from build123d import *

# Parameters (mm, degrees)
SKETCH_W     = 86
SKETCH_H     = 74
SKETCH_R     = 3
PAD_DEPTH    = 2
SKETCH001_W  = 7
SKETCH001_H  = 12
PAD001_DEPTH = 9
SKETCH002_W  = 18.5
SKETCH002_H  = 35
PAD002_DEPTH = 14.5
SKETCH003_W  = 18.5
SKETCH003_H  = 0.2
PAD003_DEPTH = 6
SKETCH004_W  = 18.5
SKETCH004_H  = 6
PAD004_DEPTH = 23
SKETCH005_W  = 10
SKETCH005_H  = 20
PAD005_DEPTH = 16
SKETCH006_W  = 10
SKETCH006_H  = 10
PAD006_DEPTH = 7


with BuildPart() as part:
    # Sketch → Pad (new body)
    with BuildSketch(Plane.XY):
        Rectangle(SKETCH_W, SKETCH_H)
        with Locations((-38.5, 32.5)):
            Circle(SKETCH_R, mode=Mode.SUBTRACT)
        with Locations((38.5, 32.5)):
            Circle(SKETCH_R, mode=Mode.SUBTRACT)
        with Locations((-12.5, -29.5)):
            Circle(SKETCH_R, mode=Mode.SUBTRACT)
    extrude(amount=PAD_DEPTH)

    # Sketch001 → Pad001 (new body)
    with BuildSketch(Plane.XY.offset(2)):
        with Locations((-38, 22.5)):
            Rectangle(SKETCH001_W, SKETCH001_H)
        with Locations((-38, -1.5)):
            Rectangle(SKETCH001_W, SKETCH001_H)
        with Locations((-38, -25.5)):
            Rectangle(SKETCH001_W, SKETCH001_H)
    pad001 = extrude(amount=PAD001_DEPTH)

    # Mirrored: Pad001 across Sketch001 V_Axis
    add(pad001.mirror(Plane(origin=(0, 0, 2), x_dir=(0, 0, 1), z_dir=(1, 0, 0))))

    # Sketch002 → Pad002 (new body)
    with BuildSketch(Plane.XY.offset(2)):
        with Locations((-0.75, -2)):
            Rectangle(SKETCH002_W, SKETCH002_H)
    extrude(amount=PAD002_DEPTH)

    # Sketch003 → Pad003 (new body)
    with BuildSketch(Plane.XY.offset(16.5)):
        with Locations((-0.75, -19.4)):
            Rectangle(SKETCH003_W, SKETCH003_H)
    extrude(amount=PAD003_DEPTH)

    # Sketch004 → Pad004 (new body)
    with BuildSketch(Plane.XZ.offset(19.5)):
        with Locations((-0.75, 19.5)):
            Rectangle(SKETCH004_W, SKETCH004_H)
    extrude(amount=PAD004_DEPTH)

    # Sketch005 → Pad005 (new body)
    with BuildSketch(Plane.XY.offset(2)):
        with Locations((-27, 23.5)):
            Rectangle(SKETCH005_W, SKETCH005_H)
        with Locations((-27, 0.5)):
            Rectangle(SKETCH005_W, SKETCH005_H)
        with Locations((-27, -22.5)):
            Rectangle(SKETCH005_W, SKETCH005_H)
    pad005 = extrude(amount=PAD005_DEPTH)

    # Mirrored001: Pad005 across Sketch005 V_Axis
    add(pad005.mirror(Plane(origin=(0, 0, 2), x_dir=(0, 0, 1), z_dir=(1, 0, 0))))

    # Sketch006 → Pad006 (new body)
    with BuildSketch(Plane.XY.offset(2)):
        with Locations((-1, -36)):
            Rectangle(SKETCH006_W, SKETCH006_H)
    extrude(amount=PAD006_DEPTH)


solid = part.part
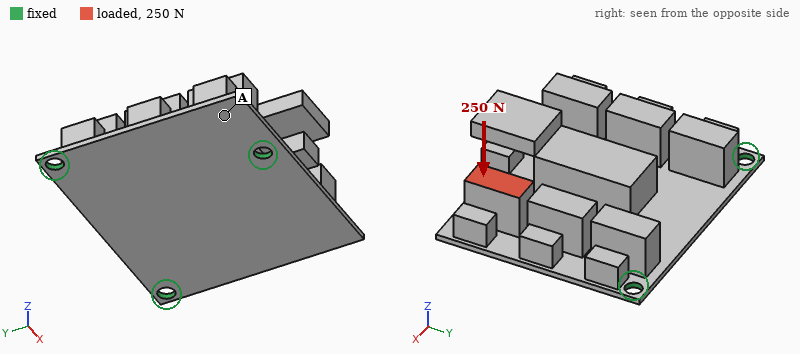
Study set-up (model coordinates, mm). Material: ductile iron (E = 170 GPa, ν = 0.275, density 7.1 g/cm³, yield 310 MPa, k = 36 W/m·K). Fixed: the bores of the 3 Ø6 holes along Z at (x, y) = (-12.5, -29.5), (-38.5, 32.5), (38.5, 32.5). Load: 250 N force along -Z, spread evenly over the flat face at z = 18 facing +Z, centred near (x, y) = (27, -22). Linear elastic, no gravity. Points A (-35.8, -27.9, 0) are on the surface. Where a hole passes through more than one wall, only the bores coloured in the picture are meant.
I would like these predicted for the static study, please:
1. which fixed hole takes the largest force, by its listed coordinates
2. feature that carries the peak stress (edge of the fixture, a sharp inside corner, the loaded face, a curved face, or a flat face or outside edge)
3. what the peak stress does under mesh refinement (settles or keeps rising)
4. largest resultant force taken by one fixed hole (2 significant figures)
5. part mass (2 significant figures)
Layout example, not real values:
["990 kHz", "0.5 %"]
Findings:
["(-12.5, -29.5)", "edge of the fixture", "keeps rising", "230 N", "350 g"]
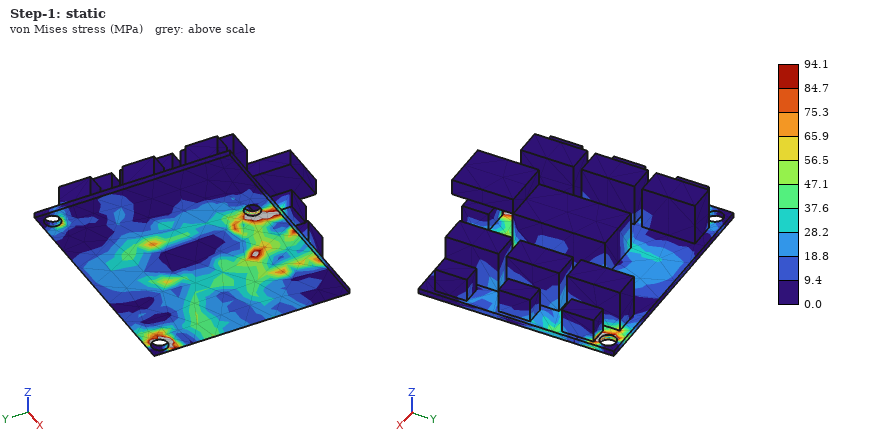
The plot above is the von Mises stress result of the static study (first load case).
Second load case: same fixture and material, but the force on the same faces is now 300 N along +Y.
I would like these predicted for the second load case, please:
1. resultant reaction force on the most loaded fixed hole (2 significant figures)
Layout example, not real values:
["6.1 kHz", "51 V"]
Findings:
["160 N"]
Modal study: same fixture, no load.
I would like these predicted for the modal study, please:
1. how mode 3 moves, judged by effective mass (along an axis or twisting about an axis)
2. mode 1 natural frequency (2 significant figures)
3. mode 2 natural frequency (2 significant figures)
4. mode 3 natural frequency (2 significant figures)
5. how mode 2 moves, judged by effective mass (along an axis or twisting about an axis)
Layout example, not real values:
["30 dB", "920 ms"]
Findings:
["along Z", "650 Hz", "850 Hz", "1200 Hz", "along Z"]
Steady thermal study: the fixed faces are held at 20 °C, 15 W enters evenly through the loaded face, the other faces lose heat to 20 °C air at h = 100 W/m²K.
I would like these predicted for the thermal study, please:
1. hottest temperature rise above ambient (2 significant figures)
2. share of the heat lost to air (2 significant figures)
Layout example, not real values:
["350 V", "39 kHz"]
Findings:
["61 K", "93 %"]
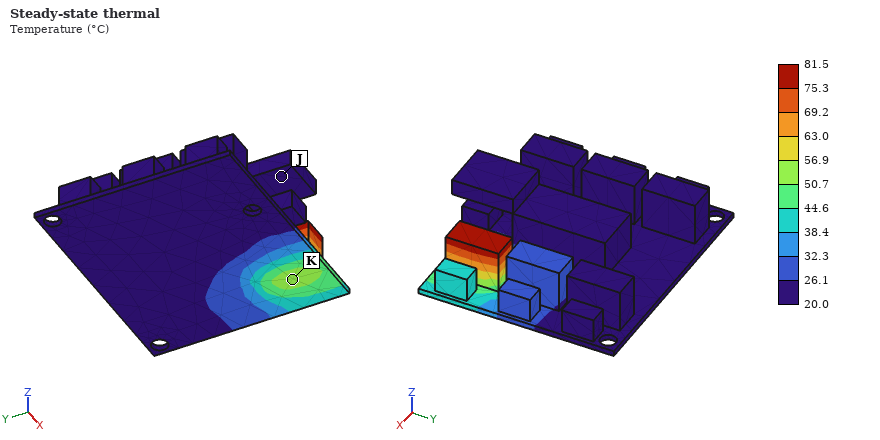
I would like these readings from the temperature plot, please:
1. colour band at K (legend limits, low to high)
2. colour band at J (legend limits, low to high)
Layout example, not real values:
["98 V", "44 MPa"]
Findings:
["50.7 to 56.9 °C", "20.0 to 26.1 °C"]
